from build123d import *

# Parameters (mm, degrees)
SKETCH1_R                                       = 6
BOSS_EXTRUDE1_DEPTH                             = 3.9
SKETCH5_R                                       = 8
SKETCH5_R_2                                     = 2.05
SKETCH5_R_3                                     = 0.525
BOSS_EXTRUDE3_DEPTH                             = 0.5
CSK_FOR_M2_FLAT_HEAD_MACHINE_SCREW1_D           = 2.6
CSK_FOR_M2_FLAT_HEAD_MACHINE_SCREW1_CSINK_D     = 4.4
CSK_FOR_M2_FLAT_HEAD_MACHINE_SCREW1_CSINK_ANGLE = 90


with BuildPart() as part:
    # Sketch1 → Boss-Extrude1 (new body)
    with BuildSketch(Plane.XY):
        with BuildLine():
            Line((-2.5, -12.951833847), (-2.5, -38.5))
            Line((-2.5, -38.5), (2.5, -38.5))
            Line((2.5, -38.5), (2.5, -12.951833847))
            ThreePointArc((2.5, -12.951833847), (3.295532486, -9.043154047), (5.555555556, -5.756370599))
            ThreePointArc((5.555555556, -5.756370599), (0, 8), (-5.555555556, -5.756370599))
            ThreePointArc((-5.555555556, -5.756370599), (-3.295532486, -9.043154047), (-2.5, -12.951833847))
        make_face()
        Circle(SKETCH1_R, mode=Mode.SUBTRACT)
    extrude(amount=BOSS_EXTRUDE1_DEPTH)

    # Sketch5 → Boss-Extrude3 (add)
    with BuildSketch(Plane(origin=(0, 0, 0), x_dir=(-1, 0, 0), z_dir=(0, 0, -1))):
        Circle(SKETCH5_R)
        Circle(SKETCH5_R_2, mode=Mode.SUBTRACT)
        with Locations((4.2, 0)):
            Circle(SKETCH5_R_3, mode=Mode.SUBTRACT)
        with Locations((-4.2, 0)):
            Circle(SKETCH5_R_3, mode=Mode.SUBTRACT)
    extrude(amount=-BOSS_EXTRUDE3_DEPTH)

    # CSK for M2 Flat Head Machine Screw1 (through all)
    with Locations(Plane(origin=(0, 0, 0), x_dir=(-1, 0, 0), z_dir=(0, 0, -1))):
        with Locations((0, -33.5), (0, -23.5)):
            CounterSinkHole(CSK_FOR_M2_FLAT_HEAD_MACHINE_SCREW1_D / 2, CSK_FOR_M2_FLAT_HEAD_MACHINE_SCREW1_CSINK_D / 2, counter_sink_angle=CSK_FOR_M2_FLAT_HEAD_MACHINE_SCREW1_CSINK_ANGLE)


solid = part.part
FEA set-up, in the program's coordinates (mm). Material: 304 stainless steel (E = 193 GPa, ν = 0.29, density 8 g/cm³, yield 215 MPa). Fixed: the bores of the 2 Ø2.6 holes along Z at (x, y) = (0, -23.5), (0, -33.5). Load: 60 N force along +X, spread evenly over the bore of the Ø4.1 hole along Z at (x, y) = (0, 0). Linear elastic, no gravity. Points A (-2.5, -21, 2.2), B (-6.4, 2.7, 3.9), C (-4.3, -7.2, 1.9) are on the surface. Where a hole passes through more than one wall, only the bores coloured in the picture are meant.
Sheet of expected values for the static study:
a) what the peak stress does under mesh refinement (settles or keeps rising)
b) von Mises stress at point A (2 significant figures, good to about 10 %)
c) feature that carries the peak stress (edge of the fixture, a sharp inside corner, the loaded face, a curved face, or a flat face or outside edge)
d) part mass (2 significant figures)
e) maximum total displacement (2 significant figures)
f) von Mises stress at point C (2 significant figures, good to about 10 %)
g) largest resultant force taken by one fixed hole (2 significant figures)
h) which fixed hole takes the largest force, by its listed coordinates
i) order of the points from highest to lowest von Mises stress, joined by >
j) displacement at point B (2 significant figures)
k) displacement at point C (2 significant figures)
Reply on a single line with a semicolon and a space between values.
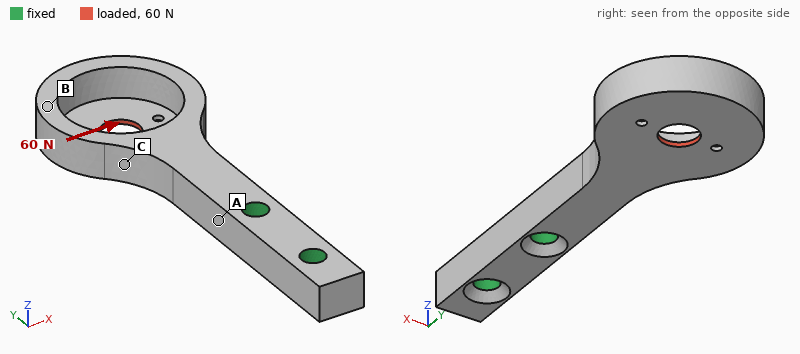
keeps rising; 80 MPa; edge of the fixture; 7.7 g; 52 µm; 17 MPa; 88 N; (0, -23.5); A > C > B; 43 µm; 22 µm
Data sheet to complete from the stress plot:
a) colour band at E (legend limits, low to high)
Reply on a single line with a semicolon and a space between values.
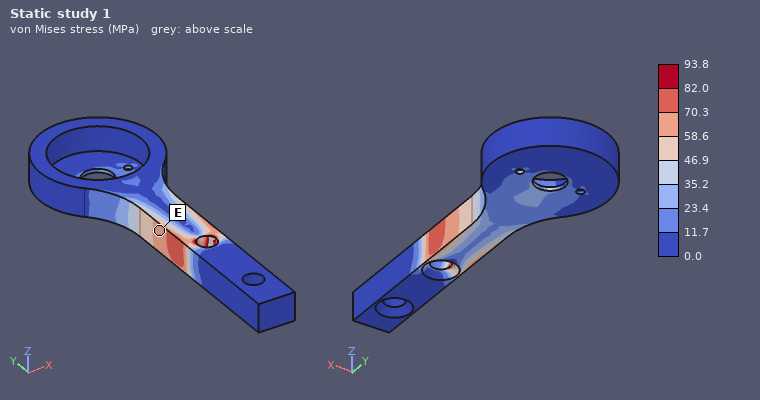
58.6 to 70.3 MPa
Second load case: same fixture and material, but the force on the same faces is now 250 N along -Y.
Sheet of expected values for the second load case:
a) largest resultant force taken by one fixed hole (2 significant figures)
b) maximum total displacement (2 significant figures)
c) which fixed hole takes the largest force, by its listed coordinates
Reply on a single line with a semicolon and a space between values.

240 N; 39 µm; (0, -23.5)
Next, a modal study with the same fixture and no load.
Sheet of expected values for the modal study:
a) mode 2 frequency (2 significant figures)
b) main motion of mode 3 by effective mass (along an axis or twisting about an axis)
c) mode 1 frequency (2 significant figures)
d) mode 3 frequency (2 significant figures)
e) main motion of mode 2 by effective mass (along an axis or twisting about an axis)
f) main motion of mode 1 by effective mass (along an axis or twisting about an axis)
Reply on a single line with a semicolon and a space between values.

3300 Hz; twisting about Y; 2700 Hz; 8200 Hz; along X; along Z
